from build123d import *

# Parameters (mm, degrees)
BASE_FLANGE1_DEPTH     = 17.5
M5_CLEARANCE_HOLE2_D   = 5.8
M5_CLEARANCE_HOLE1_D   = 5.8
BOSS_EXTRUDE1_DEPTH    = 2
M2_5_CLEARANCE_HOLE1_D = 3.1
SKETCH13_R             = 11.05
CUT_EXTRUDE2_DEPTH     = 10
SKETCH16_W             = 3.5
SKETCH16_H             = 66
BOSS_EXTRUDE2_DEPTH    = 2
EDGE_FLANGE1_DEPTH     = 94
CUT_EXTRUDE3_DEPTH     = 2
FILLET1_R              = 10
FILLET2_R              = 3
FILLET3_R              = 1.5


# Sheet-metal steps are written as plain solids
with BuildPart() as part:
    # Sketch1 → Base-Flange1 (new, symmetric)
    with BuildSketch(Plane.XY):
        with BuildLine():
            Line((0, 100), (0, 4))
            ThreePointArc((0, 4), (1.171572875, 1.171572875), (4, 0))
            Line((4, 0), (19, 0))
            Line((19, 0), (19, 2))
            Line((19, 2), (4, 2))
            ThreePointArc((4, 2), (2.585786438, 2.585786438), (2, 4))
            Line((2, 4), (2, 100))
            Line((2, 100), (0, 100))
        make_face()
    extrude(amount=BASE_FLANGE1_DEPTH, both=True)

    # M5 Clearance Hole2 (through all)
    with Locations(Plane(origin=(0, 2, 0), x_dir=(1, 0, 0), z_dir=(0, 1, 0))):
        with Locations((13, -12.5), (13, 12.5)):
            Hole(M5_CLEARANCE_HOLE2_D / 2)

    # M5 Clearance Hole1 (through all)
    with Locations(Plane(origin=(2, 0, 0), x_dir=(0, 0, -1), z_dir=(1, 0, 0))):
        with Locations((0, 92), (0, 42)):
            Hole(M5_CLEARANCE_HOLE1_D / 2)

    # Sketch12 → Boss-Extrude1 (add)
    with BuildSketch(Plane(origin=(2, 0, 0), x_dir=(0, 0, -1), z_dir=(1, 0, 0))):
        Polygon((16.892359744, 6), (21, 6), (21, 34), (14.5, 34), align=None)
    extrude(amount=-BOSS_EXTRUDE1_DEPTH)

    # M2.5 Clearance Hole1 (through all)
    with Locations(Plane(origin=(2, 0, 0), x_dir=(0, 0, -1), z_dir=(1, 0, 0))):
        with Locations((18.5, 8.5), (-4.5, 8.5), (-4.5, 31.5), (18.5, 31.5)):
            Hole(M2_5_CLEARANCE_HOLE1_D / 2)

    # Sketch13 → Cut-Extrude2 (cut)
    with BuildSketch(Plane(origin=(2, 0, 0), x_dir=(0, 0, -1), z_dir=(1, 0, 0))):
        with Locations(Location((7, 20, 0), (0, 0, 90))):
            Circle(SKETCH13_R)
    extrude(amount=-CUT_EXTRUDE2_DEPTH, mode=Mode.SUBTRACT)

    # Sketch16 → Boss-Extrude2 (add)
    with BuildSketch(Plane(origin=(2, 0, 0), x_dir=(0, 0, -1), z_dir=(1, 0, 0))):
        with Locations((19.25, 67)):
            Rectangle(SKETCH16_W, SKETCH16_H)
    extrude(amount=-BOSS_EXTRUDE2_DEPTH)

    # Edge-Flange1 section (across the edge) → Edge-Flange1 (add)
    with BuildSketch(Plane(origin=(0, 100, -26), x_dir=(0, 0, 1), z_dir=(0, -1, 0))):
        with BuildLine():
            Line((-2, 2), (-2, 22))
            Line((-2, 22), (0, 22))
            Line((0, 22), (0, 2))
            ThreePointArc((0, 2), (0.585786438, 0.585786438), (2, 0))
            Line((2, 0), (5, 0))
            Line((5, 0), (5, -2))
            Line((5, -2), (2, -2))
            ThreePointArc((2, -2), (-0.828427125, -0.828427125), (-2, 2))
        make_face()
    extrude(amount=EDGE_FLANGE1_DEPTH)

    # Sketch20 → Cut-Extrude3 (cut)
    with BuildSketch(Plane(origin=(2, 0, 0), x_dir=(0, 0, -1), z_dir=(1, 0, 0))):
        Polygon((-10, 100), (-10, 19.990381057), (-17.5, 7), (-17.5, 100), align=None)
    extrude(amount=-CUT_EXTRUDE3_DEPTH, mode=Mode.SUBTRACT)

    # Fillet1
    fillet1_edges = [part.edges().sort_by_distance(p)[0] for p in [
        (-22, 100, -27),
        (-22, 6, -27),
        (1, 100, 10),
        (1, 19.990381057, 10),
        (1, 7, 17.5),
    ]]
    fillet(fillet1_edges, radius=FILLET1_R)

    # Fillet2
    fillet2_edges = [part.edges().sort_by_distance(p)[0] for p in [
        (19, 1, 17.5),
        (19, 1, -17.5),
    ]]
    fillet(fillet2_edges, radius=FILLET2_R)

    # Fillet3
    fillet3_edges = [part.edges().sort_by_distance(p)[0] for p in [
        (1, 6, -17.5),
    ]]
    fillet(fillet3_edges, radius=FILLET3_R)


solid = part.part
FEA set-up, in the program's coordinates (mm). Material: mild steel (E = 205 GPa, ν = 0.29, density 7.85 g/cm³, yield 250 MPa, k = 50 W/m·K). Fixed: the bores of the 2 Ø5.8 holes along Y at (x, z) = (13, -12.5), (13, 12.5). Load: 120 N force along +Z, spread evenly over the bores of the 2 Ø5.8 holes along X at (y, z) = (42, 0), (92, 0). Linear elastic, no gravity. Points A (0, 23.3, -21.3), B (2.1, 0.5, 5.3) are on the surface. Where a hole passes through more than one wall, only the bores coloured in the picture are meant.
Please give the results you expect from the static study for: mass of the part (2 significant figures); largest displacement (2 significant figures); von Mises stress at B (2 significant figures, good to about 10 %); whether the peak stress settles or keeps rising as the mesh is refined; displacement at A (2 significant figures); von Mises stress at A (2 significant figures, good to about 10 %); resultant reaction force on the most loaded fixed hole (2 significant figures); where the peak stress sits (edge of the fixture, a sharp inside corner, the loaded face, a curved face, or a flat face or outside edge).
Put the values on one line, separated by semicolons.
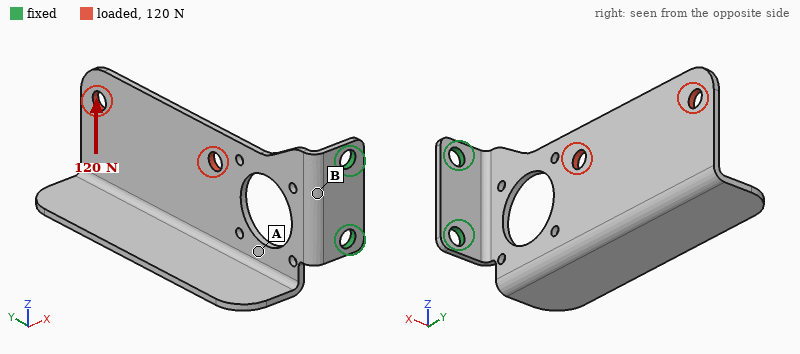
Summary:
90 g; 0.32 mm; 74 MPa; keeps rising; 0.098 mm; 20 MPa; 310 N; edge of the fixture
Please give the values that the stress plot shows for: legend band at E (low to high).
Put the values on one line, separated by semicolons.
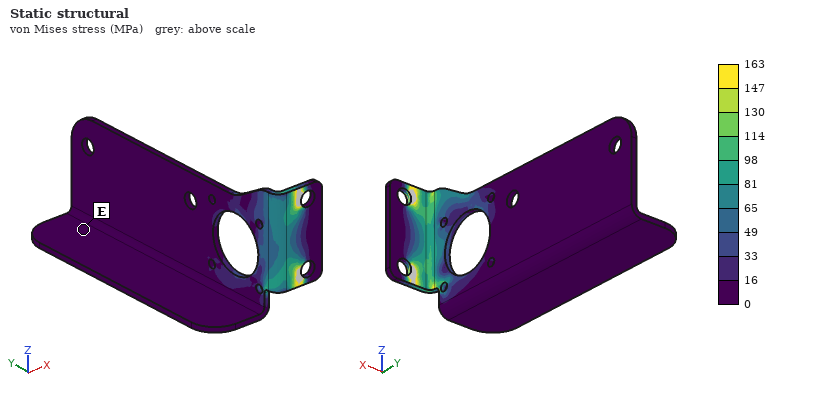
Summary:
0 to 16 MPa
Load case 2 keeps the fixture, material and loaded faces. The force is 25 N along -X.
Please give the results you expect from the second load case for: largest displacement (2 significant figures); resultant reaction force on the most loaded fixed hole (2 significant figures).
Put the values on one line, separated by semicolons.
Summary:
1.3 mm; 18 N
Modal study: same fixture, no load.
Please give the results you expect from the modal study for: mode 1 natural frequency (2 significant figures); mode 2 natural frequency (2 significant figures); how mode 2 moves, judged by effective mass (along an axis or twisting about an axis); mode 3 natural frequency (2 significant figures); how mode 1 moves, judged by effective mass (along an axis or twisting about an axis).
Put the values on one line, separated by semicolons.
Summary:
100 Hz; 480 Hz; along Z; 540 Hz; along X
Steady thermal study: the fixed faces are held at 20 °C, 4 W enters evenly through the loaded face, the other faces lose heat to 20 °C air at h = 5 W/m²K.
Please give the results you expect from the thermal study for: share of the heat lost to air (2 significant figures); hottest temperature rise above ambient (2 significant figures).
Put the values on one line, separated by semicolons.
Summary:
54 %; 60 K
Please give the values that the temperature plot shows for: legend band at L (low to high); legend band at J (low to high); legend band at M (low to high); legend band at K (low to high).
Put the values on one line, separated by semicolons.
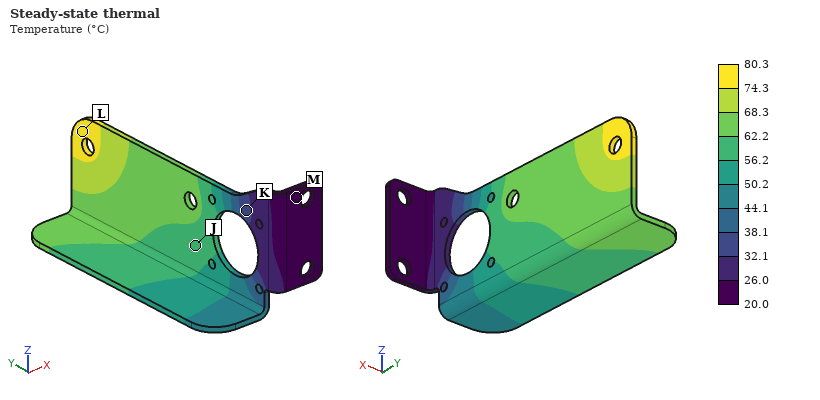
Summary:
74.3 to 80.3 °C; 56.2 to 62.2 °C; 20.0 to 26.0 °C; 32.1 to 38.1 °C
